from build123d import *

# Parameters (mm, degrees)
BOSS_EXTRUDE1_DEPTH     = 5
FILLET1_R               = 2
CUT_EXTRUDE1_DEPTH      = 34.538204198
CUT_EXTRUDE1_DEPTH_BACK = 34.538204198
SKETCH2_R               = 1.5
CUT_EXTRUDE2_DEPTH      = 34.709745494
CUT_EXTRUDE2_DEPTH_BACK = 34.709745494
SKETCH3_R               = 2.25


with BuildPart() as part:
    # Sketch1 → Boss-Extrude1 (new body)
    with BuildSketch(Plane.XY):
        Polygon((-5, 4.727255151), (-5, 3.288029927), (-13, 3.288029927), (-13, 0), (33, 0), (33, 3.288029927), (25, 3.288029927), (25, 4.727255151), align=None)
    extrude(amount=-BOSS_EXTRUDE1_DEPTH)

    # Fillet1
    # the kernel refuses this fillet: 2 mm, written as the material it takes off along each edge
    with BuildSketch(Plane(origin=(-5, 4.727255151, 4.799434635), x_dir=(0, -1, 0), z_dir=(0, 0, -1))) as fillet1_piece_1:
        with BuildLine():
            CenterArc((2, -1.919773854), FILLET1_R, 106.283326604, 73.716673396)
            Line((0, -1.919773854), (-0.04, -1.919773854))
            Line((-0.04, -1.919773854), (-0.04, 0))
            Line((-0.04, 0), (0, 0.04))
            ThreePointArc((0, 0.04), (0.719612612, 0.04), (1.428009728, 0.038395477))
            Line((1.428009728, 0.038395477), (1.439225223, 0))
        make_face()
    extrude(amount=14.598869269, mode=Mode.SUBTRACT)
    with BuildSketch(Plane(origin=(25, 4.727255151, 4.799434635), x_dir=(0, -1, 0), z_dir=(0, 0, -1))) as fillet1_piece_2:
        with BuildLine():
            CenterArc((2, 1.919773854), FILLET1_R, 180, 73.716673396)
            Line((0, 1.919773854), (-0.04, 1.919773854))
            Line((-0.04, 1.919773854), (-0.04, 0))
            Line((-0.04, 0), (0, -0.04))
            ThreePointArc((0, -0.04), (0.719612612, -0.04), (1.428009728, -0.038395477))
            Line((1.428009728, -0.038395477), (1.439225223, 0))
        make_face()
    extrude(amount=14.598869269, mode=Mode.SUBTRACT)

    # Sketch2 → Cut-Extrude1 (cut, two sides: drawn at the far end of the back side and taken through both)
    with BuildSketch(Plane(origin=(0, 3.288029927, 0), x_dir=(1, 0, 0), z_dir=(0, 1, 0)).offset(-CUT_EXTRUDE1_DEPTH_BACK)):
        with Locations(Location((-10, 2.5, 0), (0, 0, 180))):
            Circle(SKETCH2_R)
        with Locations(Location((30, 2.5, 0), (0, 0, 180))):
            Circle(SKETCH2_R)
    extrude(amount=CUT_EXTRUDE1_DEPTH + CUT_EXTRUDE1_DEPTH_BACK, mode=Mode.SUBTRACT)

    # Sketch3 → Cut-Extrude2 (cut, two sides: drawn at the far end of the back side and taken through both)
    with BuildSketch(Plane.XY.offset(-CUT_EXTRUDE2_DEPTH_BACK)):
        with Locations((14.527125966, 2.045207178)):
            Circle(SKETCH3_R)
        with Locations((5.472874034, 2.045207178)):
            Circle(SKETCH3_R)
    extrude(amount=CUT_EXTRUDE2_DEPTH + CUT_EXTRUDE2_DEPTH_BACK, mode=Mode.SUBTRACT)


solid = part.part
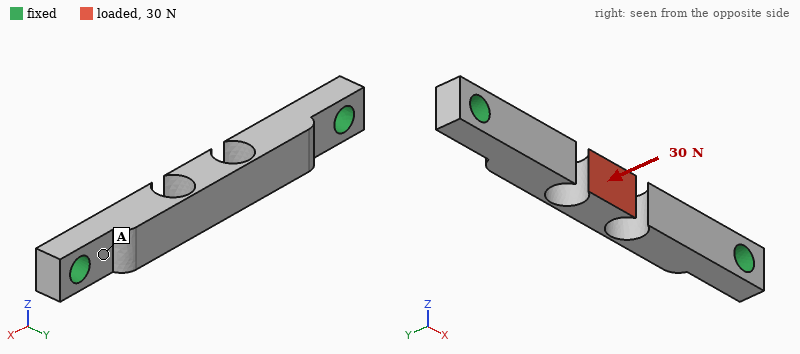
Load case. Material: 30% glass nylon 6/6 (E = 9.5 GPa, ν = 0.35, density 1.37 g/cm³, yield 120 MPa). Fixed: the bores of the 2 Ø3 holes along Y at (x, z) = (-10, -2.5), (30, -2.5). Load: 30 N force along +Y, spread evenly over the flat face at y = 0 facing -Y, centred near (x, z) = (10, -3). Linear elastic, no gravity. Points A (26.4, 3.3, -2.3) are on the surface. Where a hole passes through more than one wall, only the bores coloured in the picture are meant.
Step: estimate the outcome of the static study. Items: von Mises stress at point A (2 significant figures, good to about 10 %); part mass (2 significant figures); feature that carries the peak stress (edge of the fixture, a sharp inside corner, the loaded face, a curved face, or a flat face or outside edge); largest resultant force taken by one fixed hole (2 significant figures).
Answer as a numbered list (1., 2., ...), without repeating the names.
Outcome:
1. 8.5 MPa
2. 1.0 g
3. a curved face
4. 34 N
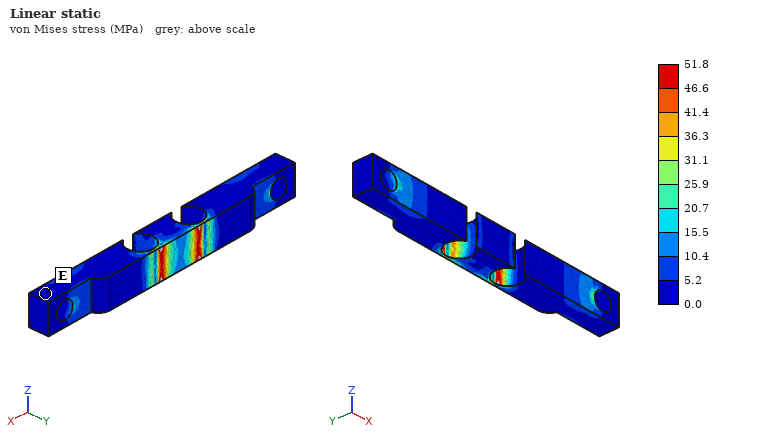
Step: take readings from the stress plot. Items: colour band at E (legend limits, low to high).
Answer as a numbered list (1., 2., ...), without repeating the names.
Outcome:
1. 0.0 to 5.2 MPa
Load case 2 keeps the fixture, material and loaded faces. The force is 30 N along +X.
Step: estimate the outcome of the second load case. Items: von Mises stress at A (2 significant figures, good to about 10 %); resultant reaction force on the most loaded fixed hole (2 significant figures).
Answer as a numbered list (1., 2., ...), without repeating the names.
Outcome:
1. 23 MPa
2. 20 N
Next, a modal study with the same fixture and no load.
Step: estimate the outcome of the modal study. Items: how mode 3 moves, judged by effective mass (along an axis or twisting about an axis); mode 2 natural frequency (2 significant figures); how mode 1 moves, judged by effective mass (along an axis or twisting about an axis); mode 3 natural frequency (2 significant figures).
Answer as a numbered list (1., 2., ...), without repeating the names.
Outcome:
1. along Y
2. 5500 Hz
3. along Z
4. 5700 Hz
